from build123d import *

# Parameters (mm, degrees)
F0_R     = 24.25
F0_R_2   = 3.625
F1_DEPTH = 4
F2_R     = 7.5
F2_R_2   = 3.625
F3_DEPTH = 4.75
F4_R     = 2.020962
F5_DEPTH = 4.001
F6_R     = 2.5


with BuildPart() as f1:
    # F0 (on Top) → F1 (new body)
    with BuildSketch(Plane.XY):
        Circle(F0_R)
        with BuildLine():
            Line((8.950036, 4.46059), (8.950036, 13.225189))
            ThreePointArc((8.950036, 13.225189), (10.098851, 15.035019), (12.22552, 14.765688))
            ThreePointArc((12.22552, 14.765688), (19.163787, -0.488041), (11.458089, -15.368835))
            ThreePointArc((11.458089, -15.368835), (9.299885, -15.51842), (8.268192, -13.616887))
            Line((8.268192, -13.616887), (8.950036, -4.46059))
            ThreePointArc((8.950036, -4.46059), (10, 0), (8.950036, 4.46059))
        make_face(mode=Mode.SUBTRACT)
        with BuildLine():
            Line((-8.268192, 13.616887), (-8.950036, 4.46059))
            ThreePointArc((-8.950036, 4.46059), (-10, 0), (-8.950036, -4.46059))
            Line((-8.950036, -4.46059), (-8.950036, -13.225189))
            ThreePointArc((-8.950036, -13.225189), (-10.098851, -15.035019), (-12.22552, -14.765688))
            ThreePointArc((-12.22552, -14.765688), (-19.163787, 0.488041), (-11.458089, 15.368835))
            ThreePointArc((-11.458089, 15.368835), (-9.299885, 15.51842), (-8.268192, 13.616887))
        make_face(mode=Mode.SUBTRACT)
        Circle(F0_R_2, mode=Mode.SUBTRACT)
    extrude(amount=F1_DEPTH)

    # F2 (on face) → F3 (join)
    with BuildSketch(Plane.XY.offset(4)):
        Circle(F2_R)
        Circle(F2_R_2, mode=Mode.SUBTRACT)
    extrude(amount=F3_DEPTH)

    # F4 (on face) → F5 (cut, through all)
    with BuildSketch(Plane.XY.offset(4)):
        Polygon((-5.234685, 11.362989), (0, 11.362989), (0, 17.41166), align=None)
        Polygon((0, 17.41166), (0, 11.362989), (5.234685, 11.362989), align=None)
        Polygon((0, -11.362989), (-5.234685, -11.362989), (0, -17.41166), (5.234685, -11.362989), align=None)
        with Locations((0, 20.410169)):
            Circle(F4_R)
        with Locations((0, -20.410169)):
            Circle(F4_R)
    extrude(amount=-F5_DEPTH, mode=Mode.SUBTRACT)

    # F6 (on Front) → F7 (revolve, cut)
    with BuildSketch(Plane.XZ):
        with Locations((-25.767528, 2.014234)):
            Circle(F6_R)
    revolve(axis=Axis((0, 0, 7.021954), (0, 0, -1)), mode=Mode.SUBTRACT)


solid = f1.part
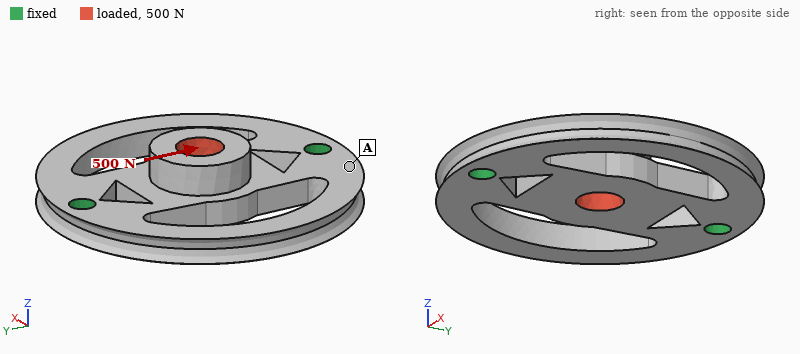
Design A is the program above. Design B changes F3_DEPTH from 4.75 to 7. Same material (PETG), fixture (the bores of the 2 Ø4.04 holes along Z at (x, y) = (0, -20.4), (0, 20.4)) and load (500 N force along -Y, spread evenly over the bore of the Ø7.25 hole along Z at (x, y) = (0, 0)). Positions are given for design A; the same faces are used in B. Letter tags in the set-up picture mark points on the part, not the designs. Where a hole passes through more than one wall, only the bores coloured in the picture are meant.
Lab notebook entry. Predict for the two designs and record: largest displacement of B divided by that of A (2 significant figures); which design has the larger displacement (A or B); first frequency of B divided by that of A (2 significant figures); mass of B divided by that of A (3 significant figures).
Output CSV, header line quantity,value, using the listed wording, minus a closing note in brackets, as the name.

quantity,value
largest displacement of B divided by that of A,1.4
which design has the larger displacement,B
first frequency of B divided by that of A,0.99
mass of B divided by that of A,1.06
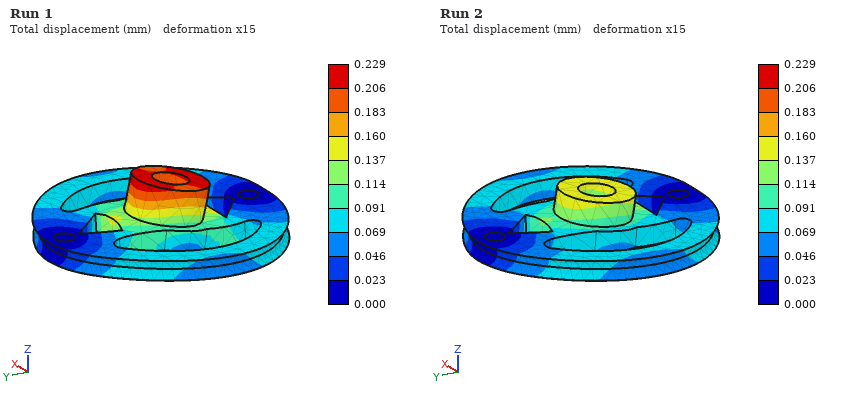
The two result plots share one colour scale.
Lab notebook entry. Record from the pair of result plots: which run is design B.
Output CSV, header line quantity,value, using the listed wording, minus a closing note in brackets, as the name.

quantity,value
which run is design B,Run 1
